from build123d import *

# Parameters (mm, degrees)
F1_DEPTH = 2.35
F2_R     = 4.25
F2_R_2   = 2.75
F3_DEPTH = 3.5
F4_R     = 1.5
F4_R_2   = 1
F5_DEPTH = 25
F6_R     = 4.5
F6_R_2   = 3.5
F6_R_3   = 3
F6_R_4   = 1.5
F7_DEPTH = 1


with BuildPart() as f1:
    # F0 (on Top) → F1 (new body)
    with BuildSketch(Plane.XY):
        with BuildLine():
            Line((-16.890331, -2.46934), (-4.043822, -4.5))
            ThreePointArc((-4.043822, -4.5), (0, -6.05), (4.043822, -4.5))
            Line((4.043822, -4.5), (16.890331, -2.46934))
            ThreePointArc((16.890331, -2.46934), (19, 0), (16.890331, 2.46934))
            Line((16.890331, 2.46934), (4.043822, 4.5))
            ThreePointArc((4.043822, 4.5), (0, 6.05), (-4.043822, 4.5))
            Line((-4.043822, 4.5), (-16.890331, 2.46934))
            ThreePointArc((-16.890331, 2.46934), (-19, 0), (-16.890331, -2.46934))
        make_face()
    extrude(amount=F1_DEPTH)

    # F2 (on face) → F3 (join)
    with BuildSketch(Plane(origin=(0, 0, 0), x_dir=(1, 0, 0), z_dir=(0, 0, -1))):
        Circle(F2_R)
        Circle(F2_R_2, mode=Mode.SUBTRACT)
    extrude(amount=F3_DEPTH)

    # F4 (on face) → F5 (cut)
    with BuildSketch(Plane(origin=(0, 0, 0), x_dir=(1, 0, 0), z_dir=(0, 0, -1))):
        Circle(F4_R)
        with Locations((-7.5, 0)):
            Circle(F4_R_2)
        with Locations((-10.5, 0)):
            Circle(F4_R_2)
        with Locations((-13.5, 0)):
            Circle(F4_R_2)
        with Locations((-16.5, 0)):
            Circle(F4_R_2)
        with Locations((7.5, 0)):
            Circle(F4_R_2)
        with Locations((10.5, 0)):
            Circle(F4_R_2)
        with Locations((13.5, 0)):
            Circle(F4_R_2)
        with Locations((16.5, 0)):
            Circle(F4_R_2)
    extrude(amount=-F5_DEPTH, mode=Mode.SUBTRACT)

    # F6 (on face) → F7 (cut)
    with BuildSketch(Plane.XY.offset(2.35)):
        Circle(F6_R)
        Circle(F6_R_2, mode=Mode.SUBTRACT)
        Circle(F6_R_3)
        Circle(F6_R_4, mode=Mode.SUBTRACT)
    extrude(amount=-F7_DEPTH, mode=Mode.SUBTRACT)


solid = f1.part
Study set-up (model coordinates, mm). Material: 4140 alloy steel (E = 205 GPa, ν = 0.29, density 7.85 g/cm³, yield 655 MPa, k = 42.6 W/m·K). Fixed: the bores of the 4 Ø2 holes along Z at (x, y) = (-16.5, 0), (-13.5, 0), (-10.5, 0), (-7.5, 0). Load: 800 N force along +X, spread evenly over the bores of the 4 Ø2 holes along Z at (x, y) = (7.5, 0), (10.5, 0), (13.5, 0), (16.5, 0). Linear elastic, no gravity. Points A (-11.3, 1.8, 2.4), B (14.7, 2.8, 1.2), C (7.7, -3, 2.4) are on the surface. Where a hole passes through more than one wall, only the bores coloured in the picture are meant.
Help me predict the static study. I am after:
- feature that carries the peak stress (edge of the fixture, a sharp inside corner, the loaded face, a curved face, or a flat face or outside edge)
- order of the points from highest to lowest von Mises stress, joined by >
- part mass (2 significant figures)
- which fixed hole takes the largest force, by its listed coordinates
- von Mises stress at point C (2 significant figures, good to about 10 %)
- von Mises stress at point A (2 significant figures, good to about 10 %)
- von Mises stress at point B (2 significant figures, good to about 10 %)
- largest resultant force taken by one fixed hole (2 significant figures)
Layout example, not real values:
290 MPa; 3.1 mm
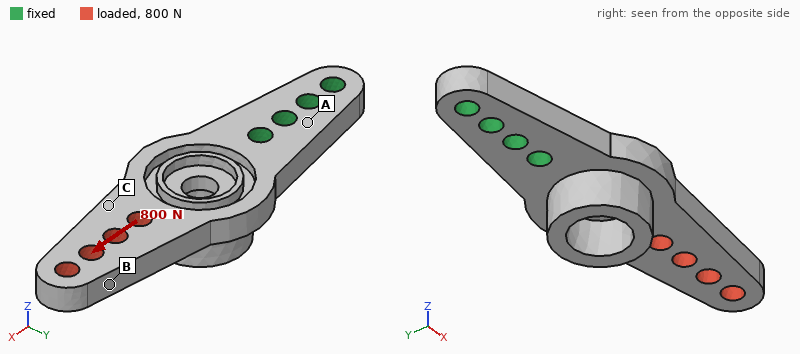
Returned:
a curved face; C > B > A; 5.2 g; (-7.5, 0); 48 MPa; 13 MPa; 24 MPa; 560 N
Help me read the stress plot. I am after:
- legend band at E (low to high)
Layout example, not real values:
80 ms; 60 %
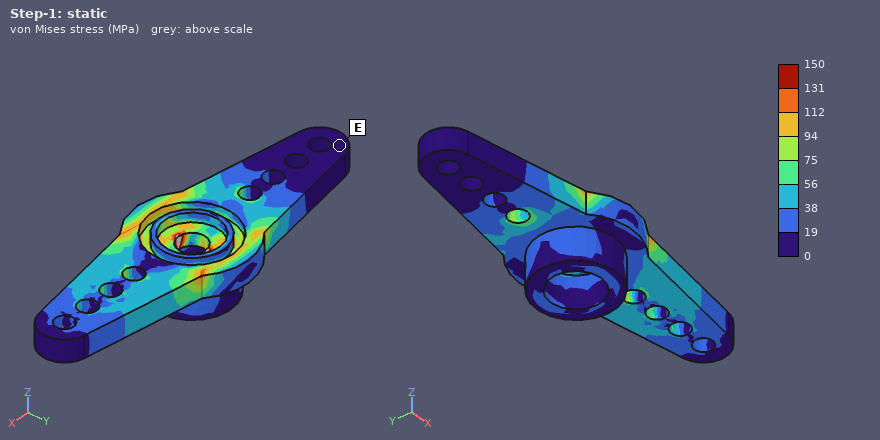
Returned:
0 to 19 MPa
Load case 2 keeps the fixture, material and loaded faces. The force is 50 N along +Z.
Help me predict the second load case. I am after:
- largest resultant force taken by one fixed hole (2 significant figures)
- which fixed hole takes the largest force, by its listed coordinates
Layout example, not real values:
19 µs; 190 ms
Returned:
130 N; (-7.5, 0)
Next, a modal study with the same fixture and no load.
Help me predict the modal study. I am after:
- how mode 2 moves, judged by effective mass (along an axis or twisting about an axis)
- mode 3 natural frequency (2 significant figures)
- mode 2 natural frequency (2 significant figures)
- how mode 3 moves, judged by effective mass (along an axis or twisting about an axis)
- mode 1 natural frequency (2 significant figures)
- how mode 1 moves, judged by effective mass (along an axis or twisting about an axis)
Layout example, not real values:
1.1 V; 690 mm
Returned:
along Y; 15 kHz; 9300 Hz; along Z; 3400 Hz; along Z
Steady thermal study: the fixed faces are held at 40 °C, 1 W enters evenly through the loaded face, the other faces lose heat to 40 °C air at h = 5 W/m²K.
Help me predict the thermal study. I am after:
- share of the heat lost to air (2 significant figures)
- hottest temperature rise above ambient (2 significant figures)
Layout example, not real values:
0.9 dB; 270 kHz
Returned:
4.6 %; 27 K
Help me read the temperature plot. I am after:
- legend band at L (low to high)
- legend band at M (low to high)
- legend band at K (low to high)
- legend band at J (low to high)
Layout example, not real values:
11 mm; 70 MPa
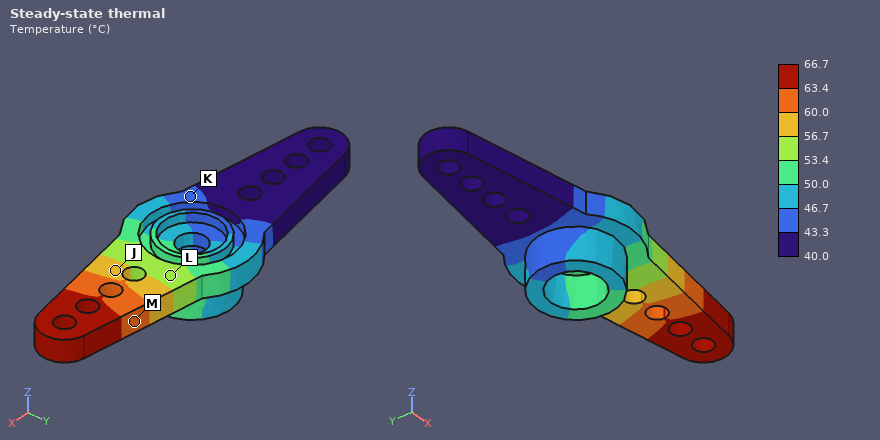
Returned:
53.4 to 56.7 °C; 60.0 to 63.4 °C; 43.3 to 46.7 °C; 56.7 to 60.0 °C
